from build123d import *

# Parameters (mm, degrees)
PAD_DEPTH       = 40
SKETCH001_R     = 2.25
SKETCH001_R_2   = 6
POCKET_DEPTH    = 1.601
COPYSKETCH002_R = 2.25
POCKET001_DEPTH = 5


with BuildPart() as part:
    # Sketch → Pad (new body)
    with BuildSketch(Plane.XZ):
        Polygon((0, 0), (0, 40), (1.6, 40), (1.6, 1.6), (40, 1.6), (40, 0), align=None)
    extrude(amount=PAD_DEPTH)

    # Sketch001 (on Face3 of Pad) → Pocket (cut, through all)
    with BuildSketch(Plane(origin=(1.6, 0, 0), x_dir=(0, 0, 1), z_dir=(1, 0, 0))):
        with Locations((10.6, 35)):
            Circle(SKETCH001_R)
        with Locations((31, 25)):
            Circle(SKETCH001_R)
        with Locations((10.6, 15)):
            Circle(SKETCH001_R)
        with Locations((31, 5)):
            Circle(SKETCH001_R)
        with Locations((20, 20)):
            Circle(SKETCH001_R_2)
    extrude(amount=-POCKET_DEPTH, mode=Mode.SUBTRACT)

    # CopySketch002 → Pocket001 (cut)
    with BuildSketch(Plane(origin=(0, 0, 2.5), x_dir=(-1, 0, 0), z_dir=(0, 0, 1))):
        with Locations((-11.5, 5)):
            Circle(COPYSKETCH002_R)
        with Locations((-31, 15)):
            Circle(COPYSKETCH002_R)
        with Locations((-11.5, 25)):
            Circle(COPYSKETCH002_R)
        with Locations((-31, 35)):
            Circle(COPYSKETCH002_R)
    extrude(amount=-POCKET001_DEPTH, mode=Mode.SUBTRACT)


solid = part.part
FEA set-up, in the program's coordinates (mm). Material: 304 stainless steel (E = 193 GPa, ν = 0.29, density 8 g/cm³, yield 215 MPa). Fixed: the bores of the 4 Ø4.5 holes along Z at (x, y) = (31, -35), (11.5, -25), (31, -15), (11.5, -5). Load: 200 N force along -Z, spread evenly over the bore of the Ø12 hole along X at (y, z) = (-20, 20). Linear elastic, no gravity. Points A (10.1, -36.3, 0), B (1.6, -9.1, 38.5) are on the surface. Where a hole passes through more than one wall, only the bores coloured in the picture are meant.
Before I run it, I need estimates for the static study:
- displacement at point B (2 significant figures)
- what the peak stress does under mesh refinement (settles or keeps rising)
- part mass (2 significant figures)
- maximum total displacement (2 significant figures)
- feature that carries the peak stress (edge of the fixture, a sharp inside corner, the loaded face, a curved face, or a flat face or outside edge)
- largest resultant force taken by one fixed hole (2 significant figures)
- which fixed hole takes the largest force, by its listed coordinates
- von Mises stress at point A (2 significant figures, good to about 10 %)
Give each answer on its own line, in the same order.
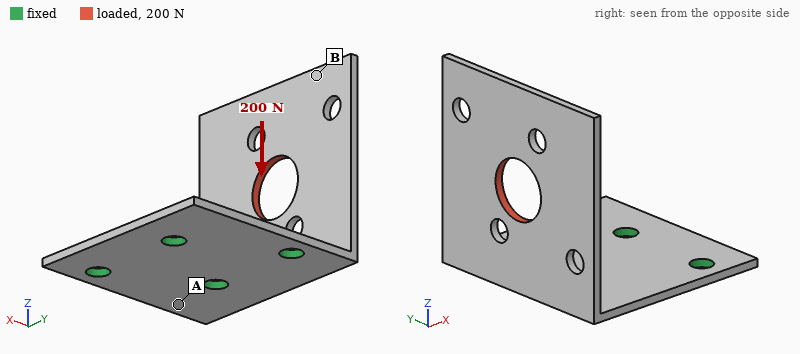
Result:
0.14 mm
keeps rising
37 g
0.15 mm
edge of the fixture
150 N
(11.5, -25)
43 MPa
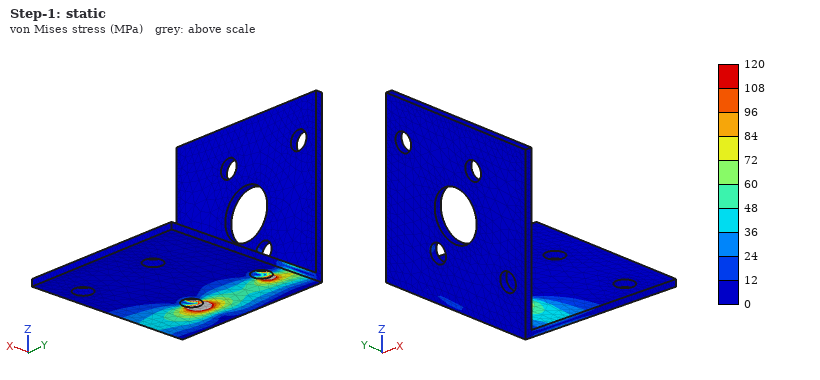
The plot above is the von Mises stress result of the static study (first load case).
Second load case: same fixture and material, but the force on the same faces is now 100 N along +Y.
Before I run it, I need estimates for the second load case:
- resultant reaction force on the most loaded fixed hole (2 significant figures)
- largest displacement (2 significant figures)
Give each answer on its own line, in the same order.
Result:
110 N
61 µm
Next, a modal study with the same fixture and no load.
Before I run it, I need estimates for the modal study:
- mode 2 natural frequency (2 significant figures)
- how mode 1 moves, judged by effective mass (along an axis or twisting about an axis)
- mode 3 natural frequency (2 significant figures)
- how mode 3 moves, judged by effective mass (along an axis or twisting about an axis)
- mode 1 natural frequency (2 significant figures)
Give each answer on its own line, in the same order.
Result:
1500 Hz
along X
2100 Hz
along Y
600 Hz
